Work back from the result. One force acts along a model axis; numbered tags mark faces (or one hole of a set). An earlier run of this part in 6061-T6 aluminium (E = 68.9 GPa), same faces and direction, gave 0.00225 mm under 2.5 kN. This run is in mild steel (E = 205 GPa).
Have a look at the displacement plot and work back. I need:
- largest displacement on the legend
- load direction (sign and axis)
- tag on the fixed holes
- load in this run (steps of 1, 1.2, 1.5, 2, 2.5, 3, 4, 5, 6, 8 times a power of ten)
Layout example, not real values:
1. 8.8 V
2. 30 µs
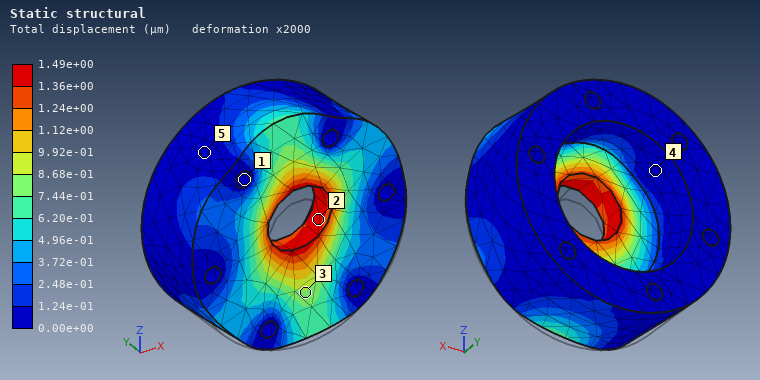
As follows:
1. 1.49e+00 µm
2. +Z
3. 1
4. 5 kN
